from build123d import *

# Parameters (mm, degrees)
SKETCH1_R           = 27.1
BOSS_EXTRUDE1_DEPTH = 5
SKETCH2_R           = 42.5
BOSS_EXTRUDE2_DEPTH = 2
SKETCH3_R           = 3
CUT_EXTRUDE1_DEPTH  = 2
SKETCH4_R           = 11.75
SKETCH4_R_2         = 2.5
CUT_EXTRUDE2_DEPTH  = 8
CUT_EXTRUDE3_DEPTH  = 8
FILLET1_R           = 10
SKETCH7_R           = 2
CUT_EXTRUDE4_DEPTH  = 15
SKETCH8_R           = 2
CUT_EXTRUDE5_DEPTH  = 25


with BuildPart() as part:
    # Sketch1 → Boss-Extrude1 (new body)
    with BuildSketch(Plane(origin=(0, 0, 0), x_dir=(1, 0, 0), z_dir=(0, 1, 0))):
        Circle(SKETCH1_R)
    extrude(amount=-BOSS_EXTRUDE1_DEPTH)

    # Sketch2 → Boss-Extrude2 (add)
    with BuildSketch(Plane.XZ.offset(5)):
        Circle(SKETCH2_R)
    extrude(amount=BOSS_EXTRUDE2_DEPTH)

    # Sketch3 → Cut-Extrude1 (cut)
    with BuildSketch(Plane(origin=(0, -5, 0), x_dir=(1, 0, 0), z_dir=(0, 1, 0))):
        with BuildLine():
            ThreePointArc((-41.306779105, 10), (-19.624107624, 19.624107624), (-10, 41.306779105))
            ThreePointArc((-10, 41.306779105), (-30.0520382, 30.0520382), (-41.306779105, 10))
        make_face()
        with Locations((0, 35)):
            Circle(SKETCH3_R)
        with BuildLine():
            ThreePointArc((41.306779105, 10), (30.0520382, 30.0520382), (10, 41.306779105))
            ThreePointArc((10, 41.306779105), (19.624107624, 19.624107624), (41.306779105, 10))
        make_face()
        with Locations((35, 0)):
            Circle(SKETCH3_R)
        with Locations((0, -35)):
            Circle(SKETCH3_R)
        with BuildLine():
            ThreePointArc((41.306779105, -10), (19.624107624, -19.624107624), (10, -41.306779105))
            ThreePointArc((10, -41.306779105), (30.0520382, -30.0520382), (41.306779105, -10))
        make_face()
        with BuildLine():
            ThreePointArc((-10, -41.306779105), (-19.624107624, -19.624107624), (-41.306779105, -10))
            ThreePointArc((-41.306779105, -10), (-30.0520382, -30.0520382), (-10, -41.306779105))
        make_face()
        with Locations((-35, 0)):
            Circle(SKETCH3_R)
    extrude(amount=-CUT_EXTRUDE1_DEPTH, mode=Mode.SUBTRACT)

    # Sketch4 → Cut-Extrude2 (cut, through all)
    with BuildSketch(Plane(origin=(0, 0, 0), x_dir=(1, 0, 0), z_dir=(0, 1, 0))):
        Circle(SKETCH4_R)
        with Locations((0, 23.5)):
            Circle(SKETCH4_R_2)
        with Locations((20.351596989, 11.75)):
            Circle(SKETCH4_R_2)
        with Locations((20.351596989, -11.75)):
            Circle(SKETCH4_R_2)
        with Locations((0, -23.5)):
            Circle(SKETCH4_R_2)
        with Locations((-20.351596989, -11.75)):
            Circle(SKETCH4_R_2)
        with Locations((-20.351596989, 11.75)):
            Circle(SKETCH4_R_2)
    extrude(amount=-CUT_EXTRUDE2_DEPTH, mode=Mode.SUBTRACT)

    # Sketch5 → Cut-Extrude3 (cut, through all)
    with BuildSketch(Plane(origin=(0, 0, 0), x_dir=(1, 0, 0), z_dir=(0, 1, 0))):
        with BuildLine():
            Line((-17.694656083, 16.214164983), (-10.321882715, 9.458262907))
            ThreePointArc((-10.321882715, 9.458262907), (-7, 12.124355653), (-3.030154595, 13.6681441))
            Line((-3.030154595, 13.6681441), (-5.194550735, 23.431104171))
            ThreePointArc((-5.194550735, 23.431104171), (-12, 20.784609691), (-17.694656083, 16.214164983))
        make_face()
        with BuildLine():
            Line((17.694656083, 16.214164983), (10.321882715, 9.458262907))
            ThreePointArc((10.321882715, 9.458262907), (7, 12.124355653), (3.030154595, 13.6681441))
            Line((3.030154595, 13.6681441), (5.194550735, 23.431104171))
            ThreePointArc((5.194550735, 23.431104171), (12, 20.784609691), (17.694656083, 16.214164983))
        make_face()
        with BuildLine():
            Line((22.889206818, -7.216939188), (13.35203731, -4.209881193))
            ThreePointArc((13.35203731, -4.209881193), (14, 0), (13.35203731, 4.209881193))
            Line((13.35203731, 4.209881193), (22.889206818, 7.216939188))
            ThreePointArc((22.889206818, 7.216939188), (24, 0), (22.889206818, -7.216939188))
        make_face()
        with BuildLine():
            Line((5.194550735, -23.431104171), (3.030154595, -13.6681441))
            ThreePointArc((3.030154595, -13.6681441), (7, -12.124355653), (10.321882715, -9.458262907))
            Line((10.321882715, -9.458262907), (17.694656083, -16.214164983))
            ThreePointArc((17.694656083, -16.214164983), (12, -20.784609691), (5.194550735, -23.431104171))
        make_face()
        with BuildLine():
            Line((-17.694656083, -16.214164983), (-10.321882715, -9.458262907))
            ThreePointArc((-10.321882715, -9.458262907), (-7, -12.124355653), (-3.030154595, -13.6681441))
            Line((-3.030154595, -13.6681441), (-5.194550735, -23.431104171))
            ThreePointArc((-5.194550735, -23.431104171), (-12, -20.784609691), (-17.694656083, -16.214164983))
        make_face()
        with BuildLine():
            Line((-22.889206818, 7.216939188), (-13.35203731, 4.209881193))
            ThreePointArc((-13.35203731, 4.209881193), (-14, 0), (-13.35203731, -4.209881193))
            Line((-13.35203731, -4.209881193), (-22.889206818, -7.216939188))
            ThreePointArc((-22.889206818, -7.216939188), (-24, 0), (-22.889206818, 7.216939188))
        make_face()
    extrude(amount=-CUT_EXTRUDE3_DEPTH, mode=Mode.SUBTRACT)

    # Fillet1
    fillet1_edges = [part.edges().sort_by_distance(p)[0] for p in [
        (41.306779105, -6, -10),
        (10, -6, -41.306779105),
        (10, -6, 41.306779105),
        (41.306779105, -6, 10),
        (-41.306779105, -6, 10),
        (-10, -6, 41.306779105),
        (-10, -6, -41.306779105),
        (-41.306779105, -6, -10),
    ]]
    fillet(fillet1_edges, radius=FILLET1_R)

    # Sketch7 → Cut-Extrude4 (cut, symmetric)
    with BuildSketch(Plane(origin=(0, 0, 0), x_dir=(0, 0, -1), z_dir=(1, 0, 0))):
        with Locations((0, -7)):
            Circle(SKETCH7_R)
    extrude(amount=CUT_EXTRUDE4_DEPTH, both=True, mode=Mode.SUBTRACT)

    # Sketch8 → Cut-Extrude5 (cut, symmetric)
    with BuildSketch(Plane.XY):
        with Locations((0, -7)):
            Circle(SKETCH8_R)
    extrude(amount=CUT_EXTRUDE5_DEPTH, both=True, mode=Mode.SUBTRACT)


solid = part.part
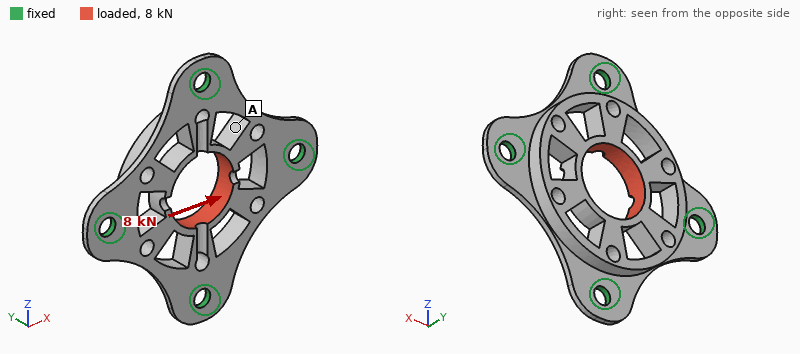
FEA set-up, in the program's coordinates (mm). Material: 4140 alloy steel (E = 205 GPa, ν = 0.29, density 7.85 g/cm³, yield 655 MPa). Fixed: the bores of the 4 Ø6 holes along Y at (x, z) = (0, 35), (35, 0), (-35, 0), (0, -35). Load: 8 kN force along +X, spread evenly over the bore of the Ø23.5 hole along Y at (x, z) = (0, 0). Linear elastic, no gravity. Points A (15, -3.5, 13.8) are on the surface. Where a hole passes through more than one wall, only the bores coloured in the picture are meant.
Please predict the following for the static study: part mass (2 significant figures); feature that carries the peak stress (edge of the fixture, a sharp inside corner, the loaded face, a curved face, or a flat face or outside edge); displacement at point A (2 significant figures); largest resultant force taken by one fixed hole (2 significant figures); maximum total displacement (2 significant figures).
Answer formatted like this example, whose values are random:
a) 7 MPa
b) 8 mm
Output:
a) 79 g
b) the loaded face
c) 9.2 µm
d) 2.9 kN
e) 22 µm
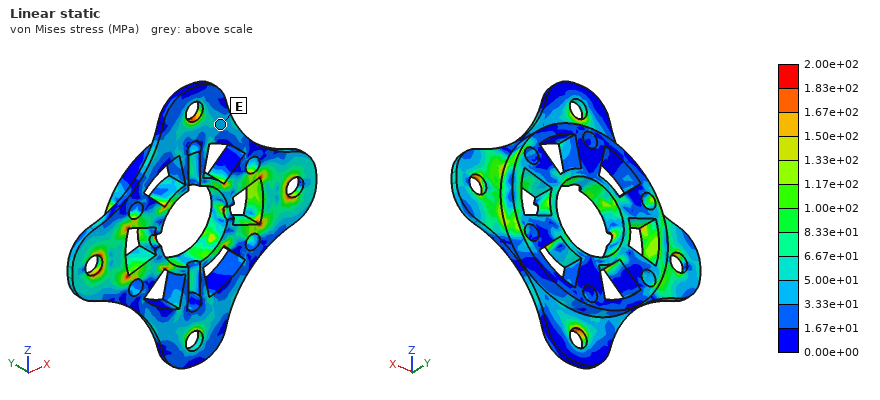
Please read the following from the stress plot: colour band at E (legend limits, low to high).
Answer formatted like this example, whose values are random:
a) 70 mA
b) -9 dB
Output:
a) 3.33e+01 to 5.00e+01 MPa
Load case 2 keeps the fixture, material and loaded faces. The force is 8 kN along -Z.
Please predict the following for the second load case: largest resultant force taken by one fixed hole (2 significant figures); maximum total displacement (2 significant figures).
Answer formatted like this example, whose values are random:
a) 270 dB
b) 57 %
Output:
a) 2.6 kN
b) 29 µm
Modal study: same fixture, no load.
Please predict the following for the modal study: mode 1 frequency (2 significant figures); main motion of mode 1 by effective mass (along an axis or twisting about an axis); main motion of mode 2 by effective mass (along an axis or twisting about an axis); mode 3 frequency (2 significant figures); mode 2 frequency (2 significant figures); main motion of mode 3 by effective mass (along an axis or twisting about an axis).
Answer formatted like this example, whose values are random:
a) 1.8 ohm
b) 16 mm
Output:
a) 6100 Hz
b) along Y
c) twisting about X
d) 8700 Hz
e) 8300 Hz
f) twisting about Z
